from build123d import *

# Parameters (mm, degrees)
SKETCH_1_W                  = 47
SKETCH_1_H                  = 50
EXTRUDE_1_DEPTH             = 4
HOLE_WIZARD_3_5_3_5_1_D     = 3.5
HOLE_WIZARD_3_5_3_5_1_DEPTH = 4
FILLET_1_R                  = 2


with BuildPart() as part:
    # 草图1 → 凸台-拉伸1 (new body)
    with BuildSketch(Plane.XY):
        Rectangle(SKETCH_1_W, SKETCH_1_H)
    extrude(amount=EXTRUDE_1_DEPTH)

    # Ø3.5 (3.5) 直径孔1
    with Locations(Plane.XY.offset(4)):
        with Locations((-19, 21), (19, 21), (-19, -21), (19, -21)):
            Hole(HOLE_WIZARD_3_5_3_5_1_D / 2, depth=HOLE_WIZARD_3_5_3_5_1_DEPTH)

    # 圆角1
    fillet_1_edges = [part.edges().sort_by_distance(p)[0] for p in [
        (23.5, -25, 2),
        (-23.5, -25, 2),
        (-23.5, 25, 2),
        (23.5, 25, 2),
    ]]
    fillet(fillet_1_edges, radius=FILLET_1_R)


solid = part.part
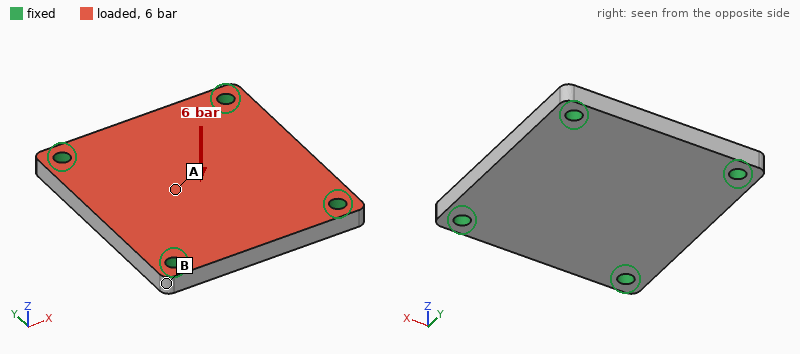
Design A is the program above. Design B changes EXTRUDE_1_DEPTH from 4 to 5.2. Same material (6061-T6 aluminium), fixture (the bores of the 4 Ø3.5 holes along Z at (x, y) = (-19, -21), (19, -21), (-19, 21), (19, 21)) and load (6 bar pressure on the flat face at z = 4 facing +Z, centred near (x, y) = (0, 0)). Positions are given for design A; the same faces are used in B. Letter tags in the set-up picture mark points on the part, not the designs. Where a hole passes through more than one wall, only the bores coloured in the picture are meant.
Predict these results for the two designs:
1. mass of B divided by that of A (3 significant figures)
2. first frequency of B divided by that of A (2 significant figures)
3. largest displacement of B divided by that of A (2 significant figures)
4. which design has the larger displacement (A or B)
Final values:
1.30
1.2
0.50
A
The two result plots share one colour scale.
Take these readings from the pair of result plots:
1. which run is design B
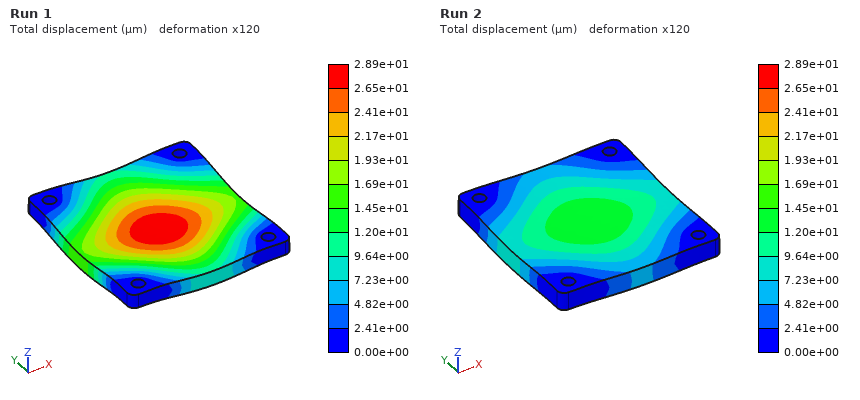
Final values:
Run 2
